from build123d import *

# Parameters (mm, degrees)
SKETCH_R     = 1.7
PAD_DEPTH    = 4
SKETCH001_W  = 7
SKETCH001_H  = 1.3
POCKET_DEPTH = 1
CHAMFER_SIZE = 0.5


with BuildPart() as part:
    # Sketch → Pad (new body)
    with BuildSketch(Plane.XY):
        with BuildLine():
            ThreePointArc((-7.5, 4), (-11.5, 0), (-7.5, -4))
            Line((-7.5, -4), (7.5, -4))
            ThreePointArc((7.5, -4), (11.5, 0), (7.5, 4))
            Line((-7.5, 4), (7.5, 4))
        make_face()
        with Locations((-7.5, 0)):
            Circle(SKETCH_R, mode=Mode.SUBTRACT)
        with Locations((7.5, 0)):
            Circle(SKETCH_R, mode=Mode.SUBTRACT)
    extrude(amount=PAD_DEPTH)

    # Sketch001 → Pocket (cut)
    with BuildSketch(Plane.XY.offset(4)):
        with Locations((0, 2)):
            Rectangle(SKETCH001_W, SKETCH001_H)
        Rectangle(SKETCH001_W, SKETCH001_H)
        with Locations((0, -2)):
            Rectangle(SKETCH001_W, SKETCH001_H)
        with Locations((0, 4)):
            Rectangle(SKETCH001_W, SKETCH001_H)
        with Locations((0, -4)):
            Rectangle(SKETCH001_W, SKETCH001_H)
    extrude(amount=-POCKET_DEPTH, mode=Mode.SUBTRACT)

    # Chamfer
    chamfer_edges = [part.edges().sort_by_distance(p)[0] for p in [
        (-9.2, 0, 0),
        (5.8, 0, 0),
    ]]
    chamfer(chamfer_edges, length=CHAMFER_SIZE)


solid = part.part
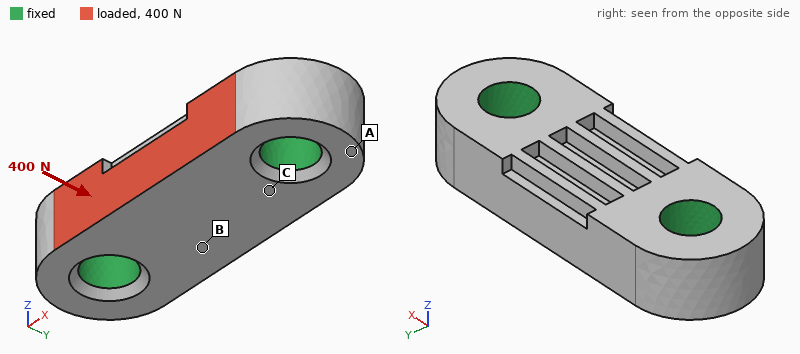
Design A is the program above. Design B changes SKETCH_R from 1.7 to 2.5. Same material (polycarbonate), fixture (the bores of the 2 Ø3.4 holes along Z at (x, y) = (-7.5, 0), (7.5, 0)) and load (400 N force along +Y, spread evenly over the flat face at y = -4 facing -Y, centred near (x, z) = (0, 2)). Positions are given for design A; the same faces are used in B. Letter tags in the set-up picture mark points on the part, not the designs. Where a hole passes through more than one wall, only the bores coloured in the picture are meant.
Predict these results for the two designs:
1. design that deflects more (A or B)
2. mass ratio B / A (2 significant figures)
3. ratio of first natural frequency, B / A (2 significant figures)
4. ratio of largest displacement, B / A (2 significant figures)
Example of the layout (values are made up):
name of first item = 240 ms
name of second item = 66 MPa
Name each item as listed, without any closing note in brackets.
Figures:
design that deflects more = A
mass ratio B / A = 0.85
ratio of first natural frequency, B / A = 1.3
ratio of largest displacement, B / A = 0.73
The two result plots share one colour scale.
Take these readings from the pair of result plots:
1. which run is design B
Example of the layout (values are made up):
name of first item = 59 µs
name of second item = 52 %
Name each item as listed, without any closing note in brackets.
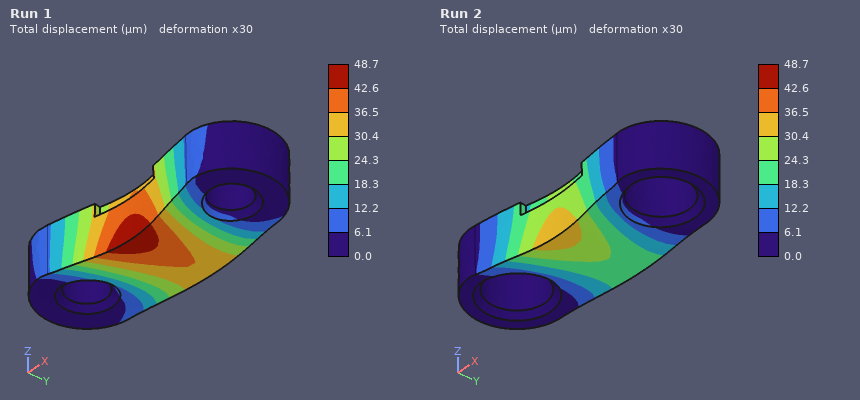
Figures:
which run is design B = Run 2
